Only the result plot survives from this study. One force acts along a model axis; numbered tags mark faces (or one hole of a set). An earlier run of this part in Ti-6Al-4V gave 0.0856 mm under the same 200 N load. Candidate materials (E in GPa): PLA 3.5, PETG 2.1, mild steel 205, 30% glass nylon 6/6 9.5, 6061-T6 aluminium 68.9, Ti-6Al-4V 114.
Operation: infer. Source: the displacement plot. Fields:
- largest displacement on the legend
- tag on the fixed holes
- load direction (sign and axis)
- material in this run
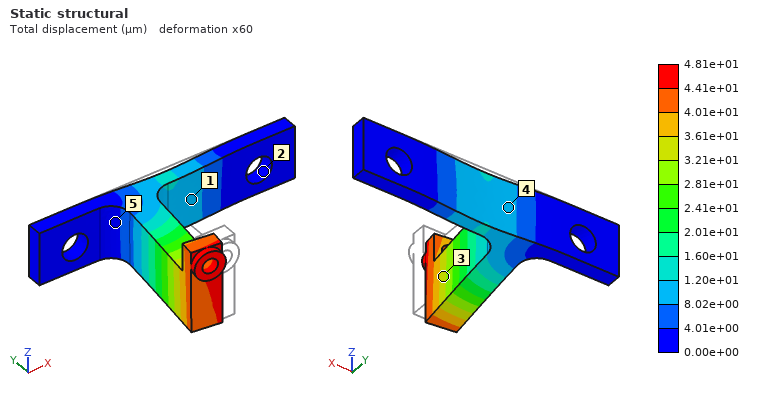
4.81e+01 µm
2
-X
mild steel
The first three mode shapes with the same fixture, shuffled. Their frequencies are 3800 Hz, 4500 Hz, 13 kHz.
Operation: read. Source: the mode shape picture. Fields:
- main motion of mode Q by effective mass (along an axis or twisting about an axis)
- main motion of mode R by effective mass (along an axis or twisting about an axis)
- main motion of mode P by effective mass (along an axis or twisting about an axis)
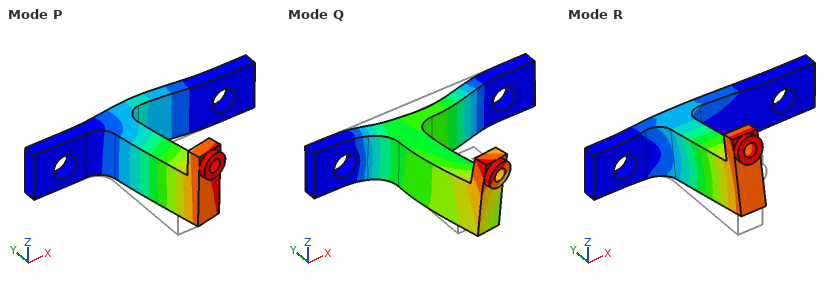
along Y
along Z
along X
